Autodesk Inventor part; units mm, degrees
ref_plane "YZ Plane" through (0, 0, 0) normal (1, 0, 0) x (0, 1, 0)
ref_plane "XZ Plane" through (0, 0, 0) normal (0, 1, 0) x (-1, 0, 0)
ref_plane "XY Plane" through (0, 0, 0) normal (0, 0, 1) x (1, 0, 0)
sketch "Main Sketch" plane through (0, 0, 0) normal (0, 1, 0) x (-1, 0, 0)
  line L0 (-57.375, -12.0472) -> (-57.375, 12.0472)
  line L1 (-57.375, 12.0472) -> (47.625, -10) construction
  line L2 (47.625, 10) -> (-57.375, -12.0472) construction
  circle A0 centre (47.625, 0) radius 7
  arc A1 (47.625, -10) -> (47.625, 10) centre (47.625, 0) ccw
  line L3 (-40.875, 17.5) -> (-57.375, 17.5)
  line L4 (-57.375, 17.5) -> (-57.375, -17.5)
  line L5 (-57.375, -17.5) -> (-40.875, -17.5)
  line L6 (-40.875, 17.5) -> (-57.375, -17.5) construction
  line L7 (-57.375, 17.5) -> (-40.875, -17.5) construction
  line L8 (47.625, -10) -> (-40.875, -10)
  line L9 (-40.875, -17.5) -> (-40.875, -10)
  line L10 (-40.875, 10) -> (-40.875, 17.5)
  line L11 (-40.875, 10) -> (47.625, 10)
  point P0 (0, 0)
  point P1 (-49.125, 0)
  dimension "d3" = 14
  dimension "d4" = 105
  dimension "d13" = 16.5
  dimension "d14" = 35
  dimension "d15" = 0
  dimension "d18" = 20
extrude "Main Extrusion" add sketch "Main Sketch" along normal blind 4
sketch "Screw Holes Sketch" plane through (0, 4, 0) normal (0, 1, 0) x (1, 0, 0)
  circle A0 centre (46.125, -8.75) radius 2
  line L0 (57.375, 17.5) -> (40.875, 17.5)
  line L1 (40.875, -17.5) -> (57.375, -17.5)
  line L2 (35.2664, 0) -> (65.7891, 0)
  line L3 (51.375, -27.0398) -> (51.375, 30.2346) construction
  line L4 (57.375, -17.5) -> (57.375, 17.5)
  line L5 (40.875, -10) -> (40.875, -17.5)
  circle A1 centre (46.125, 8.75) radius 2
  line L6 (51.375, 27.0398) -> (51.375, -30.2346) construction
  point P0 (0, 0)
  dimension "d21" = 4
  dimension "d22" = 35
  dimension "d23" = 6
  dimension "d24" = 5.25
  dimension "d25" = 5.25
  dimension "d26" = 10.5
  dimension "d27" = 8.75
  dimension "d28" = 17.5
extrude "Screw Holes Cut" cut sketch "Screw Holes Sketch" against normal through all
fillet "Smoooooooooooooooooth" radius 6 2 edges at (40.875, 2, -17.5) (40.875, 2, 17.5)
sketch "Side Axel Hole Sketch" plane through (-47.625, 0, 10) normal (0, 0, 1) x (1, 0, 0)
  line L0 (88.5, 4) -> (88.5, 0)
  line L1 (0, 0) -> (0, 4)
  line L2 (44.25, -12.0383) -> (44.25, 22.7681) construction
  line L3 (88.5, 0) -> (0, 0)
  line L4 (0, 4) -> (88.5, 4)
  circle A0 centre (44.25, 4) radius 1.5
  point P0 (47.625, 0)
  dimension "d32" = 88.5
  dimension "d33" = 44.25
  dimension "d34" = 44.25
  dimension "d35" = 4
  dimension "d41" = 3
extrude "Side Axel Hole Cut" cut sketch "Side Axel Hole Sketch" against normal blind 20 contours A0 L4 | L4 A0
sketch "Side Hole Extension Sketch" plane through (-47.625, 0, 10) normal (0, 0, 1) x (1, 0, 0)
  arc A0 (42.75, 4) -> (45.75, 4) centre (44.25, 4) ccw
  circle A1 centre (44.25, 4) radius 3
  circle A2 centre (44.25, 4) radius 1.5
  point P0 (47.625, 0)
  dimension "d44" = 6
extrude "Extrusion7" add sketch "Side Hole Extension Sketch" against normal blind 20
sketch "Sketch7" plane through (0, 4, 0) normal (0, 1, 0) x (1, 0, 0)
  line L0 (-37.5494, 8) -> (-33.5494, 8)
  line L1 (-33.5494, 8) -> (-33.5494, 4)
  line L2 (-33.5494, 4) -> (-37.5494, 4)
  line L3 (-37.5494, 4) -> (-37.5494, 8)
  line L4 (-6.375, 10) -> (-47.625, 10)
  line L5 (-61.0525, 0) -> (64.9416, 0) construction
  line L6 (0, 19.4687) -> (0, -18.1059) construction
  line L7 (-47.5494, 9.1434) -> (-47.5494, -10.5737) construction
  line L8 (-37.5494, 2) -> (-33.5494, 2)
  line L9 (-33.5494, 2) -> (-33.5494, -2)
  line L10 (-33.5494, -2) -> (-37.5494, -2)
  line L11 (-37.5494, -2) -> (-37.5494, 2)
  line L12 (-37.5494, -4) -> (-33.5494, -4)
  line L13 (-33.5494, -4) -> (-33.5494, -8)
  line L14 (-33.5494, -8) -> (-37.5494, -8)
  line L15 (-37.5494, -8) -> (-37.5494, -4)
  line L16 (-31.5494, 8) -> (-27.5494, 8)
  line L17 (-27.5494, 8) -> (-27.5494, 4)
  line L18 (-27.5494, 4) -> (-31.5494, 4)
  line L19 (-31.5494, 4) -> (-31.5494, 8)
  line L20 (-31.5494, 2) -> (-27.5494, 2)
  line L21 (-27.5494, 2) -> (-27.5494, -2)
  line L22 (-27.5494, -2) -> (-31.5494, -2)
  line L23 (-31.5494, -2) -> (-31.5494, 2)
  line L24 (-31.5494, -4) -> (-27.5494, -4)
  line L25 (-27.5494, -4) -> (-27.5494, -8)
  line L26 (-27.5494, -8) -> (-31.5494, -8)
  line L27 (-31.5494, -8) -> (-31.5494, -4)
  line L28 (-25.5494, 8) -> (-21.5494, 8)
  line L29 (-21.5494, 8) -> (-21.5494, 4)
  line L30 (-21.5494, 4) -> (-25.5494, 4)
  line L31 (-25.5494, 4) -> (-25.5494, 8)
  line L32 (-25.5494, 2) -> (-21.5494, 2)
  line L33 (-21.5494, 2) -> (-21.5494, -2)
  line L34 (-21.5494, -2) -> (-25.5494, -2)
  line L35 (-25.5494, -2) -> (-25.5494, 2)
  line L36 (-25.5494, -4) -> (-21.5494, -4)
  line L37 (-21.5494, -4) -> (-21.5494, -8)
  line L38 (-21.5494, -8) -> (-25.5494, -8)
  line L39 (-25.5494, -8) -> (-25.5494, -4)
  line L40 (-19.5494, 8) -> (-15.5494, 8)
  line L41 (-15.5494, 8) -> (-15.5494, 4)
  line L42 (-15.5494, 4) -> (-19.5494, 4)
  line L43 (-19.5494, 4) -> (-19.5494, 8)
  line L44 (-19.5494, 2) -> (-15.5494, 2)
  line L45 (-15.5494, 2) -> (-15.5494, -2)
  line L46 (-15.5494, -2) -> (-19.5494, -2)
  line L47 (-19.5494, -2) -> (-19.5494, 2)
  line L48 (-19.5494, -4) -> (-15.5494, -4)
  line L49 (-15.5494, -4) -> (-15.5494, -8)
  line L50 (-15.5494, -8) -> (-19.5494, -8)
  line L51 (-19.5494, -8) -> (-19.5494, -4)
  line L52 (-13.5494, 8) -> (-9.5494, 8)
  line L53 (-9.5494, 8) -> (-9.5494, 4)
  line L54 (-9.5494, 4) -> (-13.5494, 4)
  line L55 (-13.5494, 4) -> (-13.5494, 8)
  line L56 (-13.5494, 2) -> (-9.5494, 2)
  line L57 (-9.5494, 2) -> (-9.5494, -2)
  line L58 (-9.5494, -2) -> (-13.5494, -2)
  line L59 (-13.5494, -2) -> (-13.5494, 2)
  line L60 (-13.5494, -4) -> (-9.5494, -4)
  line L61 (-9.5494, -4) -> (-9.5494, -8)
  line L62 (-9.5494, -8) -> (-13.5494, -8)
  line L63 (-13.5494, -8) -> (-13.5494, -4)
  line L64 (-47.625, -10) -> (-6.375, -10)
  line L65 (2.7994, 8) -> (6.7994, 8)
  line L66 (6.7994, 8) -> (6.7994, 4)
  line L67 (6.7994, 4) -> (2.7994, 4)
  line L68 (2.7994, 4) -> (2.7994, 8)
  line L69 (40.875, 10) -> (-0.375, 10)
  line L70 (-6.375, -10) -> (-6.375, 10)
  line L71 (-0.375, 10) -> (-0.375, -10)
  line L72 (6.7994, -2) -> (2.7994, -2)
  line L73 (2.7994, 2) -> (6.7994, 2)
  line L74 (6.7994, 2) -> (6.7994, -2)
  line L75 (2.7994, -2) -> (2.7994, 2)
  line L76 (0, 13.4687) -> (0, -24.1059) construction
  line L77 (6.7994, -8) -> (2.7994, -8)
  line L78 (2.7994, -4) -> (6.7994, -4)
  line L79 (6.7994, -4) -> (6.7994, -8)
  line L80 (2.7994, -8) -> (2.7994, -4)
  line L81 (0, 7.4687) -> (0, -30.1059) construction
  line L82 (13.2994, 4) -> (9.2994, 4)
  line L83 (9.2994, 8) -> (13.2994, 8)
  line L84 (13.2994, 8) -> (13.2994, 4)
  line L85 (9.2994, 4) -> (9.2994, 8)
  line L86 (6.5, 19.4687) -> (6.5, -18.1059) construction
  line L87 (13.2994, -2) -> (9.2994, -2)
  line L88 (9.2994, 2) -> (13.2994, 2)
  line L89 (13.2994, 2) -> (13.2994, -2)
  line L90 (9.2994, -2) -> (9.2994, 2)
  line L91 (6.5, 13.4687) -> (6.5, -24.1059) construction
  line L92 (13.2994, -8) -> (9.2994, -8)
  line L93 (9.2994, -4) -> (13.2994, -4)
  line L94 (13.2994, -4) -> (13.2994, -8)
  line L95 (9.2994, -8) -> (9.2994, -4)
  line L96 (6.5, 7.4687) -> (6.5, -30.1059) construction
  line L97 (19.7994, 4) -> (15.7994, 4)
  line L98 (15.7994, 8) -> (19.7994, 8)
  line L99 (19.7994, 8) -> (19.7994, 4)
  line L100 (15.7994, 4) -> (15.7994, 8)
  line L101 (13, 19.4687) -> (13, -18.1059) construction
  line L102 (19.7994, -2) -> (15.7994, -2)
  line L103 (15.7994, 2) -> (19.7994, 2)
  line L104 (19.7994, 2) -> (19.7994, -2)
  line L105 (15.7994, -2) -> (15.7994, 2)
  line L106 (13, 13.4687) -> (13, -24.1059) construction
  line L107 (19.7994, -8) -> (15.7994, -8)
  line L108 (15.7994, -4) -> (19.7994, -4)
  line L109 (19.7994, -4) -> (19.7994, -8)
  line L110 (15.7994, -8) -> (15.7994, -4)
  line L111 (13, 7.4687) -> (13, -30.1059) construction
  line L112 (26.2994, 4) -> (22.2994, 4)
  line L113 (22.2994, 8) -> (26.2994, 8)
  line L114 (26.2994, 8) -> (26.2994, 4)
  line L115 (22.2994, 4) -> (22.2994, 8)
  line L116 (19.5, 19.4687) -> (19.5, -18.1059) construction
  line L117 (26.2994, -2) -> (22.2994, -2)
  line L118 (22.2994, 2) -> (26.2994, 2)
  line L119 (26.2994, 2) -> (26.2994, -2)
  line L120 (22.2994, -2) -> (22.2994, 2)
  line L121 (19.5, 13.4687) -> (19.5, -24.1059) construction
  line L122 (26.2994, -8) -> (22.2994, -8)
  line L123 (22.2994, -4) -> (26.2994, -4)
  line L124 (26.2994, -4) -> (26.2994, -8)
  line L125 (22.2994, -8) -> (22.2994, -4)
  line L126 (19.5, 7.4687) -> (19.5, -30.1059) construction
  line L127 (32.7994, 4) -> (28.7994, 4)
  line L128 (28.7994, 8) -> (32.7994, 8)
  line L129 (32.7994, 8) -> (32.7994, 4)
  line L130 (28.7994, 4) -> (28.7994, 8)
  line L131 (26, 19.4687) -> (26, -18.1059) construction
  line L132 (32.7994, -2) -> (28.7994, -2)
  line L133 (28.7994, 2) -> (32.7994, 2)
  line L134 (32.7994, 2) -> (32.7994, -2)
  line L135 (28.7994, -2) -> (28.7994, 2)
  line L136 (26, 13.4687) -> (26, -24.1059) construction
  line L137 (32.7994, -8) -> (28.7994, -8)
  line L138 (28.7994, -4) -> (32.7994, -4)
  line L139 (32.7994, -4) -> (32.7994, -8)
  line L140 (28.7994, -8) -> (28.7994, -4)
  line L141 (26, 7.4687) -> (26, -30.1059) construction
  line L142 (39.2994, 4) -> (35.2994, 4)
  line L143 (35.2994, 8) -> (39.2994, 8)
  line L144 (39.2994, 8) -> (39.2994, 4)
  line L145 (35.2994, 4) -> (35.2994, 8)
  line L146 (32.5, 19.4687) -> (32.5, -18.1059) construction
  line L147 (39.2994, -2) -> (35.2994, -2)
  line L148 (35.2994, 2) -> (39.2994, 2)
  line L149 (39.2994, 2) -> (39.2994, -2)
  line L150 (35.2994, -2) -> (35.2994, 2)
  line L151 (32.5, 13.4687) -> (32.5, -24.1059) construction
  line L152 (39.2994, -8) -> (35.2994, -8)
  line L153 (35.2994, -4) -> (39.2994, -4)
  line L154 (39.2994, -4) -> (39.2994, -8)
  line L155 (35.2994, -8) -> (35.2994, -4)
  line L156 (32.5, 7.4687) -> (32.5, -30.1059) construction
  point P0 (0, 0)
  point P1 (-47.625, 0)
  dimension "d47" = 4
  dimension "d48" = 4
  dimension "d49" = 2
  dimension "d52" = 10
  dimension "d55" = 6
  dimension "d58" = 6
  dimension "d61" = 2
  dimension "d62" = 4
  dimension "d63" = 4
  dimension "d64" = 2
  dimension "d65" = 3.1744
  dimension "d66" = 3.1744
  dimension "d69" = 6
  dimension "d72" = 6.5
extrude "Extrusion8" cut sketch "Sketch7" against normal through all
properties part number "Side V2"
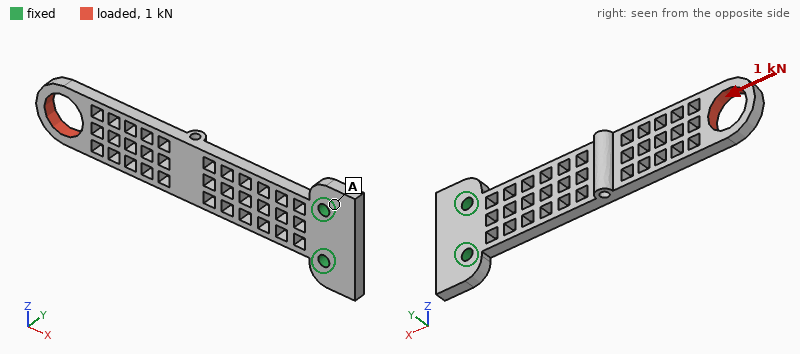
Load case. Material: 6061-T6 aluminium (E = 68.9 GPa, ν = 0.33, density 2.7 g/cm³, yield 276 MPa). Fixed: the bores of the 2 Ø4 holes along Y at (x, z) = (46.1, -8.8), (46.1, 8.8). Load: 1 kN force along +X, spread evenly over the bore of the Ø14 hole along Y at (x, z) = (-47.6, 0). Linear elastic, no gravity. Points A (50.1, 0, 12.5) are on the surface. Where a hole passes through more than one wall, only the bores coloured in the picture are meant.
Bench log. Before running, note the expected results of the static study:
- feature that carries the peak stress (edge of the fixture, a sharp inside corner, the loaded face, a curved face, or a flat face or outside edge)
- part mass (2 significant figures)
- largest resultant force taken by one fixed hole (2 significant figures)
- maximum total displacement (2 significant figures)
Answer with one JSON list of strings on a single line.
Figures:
["the loaded face", "20 g", "510 N", "51 µm"]
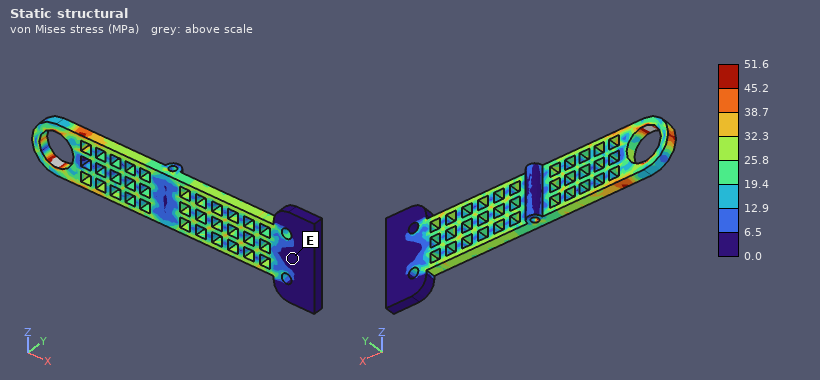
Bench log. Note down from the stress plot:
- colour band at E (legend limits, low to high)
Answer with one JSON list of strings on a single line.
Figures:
["0.0 to 6.5 MPa"]
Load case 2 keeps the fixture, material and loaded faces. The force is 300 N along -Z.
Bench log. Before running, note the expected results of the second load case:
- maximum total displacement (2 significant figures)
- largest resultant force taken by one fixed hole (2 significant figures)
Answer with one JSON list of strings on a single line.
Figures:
["0.93 mm", "1.6 kN"]
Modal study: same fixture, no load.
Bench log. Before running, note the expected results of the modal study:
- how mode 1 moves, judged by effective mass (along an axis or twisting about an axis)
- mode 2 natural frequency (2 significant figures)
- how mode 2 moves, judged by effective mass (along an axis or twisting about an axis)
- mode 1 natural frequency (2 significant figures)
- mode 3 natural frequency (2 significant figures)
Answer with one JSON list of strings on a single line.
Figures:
["along Y", "1500 Hz", "along Z", "300 Hz", "1700 Hz"]
